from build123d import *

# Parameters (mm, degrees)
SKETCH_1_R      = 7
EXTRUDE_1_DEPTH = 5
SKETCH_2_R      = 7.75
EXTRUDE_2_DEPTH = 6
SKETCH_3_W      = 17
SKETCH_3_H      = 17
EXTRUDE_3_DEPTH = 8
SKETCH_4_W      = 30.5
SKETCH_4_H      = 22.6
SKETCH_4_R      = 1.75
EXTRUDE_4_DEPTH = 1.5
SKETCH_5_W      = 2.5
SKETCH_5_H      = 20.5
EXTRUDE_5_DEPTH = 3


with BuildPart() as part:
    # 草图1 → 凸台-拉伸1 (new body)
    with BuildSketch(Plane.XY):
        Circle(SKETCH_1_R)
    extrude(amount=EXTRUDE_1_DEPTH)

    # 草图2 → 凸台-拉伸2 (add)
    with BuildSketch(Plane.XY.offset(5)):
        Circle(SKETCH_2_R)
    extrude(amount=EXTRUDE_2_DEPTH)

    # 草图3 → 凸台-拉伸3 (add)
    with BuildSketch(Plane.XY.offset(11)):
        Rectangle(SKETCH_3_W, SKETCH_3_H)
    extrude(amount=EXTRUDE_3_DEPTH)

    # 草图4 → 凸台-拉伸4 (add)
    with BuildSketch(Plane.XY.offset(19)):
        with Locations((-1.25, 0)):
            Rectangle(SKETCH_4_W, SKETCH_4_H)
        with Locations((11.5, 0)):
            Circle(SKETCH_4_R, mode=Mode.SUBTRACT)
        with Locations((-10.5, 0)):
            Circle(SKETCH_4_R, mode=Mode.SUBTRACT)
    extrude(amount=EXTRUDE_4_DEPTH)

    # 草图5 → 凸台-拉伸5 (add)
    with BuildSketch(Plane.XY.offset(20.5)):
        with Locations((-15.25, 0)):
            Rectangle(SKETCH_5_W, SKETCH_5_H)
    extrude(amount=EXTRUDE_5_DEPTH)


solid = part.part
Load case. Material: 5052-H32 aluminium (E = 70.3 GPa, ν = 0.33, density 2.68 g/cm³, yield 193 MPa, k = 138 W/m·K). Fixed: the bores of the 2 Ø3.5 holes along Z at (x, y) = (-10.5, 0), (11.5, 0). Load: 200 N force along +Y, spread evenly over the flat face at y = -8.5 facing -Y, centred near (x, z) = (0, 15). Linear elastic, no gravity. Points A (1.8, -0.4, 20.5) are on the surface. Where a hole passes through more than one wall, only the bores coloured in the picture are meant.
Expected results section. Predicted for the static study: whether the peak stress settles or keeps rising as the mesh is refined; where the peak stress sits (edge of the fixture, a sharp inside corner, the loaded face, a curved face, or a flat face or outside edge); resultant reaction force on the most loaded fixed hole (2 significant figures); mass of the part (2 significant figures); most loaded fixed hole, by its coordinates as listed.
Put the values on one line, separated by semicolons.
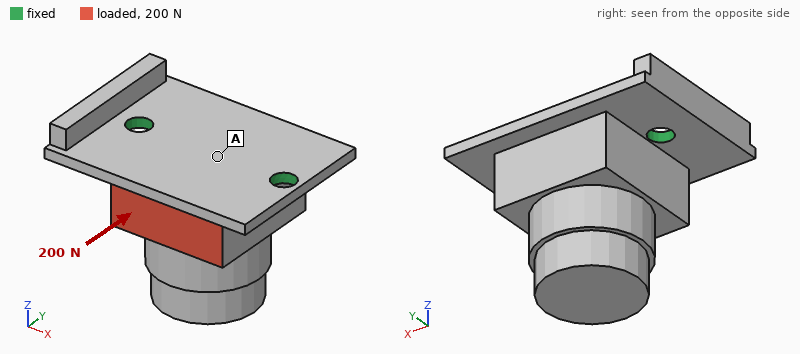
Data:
keeps rising; edge of the fixture; 110 N; 14 g; (-10.5, 0)
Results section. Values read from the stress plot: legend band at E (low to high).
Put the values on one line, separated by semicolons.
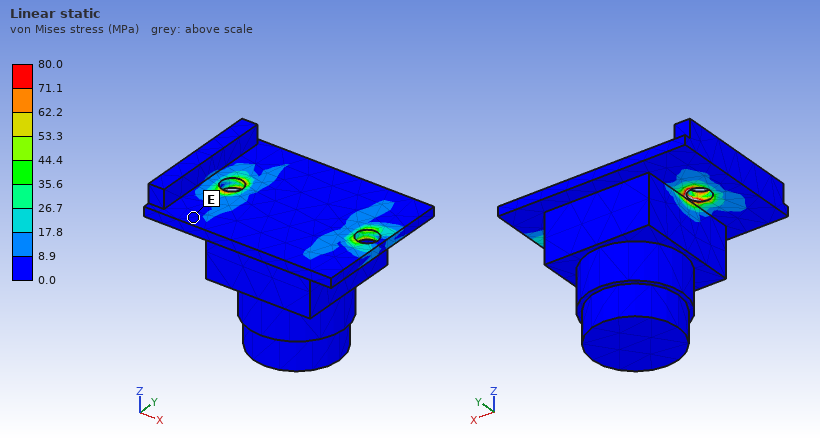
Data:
0.0 to 8.9 MPa
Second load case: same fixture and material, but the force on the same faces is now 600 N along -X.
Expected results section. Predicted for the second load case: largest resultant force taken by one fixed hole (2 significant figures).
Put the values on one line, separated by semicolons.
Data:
430 N
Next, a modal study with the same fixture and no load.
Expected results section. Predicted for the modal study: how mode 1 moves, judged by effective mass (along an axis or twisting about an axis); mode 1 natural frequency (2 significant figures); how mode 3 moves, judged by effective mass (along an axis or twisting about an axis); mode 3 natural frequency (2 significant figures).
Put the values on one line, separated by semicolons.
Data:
along Y; 3500 Hz; along Z; 18 kHz
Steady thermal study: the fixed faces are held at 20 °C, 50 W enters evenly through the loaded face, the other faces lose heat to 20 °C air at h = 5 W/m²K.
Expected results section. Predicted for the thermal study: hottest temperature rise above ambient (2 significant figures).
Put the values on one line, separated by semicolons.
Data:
49 K
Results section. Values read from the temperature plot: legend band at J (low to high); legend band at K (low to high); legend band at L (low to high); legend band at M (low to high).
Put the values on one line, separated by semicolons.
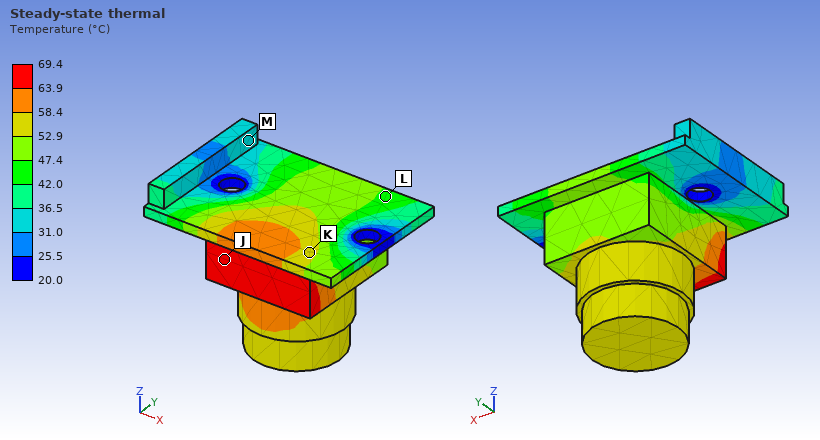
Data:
63.9 to 69.4 °C; 52.9 to 58.4 °C; 42.0 to 47.4 °C; 31.0 to 36.5 °C
